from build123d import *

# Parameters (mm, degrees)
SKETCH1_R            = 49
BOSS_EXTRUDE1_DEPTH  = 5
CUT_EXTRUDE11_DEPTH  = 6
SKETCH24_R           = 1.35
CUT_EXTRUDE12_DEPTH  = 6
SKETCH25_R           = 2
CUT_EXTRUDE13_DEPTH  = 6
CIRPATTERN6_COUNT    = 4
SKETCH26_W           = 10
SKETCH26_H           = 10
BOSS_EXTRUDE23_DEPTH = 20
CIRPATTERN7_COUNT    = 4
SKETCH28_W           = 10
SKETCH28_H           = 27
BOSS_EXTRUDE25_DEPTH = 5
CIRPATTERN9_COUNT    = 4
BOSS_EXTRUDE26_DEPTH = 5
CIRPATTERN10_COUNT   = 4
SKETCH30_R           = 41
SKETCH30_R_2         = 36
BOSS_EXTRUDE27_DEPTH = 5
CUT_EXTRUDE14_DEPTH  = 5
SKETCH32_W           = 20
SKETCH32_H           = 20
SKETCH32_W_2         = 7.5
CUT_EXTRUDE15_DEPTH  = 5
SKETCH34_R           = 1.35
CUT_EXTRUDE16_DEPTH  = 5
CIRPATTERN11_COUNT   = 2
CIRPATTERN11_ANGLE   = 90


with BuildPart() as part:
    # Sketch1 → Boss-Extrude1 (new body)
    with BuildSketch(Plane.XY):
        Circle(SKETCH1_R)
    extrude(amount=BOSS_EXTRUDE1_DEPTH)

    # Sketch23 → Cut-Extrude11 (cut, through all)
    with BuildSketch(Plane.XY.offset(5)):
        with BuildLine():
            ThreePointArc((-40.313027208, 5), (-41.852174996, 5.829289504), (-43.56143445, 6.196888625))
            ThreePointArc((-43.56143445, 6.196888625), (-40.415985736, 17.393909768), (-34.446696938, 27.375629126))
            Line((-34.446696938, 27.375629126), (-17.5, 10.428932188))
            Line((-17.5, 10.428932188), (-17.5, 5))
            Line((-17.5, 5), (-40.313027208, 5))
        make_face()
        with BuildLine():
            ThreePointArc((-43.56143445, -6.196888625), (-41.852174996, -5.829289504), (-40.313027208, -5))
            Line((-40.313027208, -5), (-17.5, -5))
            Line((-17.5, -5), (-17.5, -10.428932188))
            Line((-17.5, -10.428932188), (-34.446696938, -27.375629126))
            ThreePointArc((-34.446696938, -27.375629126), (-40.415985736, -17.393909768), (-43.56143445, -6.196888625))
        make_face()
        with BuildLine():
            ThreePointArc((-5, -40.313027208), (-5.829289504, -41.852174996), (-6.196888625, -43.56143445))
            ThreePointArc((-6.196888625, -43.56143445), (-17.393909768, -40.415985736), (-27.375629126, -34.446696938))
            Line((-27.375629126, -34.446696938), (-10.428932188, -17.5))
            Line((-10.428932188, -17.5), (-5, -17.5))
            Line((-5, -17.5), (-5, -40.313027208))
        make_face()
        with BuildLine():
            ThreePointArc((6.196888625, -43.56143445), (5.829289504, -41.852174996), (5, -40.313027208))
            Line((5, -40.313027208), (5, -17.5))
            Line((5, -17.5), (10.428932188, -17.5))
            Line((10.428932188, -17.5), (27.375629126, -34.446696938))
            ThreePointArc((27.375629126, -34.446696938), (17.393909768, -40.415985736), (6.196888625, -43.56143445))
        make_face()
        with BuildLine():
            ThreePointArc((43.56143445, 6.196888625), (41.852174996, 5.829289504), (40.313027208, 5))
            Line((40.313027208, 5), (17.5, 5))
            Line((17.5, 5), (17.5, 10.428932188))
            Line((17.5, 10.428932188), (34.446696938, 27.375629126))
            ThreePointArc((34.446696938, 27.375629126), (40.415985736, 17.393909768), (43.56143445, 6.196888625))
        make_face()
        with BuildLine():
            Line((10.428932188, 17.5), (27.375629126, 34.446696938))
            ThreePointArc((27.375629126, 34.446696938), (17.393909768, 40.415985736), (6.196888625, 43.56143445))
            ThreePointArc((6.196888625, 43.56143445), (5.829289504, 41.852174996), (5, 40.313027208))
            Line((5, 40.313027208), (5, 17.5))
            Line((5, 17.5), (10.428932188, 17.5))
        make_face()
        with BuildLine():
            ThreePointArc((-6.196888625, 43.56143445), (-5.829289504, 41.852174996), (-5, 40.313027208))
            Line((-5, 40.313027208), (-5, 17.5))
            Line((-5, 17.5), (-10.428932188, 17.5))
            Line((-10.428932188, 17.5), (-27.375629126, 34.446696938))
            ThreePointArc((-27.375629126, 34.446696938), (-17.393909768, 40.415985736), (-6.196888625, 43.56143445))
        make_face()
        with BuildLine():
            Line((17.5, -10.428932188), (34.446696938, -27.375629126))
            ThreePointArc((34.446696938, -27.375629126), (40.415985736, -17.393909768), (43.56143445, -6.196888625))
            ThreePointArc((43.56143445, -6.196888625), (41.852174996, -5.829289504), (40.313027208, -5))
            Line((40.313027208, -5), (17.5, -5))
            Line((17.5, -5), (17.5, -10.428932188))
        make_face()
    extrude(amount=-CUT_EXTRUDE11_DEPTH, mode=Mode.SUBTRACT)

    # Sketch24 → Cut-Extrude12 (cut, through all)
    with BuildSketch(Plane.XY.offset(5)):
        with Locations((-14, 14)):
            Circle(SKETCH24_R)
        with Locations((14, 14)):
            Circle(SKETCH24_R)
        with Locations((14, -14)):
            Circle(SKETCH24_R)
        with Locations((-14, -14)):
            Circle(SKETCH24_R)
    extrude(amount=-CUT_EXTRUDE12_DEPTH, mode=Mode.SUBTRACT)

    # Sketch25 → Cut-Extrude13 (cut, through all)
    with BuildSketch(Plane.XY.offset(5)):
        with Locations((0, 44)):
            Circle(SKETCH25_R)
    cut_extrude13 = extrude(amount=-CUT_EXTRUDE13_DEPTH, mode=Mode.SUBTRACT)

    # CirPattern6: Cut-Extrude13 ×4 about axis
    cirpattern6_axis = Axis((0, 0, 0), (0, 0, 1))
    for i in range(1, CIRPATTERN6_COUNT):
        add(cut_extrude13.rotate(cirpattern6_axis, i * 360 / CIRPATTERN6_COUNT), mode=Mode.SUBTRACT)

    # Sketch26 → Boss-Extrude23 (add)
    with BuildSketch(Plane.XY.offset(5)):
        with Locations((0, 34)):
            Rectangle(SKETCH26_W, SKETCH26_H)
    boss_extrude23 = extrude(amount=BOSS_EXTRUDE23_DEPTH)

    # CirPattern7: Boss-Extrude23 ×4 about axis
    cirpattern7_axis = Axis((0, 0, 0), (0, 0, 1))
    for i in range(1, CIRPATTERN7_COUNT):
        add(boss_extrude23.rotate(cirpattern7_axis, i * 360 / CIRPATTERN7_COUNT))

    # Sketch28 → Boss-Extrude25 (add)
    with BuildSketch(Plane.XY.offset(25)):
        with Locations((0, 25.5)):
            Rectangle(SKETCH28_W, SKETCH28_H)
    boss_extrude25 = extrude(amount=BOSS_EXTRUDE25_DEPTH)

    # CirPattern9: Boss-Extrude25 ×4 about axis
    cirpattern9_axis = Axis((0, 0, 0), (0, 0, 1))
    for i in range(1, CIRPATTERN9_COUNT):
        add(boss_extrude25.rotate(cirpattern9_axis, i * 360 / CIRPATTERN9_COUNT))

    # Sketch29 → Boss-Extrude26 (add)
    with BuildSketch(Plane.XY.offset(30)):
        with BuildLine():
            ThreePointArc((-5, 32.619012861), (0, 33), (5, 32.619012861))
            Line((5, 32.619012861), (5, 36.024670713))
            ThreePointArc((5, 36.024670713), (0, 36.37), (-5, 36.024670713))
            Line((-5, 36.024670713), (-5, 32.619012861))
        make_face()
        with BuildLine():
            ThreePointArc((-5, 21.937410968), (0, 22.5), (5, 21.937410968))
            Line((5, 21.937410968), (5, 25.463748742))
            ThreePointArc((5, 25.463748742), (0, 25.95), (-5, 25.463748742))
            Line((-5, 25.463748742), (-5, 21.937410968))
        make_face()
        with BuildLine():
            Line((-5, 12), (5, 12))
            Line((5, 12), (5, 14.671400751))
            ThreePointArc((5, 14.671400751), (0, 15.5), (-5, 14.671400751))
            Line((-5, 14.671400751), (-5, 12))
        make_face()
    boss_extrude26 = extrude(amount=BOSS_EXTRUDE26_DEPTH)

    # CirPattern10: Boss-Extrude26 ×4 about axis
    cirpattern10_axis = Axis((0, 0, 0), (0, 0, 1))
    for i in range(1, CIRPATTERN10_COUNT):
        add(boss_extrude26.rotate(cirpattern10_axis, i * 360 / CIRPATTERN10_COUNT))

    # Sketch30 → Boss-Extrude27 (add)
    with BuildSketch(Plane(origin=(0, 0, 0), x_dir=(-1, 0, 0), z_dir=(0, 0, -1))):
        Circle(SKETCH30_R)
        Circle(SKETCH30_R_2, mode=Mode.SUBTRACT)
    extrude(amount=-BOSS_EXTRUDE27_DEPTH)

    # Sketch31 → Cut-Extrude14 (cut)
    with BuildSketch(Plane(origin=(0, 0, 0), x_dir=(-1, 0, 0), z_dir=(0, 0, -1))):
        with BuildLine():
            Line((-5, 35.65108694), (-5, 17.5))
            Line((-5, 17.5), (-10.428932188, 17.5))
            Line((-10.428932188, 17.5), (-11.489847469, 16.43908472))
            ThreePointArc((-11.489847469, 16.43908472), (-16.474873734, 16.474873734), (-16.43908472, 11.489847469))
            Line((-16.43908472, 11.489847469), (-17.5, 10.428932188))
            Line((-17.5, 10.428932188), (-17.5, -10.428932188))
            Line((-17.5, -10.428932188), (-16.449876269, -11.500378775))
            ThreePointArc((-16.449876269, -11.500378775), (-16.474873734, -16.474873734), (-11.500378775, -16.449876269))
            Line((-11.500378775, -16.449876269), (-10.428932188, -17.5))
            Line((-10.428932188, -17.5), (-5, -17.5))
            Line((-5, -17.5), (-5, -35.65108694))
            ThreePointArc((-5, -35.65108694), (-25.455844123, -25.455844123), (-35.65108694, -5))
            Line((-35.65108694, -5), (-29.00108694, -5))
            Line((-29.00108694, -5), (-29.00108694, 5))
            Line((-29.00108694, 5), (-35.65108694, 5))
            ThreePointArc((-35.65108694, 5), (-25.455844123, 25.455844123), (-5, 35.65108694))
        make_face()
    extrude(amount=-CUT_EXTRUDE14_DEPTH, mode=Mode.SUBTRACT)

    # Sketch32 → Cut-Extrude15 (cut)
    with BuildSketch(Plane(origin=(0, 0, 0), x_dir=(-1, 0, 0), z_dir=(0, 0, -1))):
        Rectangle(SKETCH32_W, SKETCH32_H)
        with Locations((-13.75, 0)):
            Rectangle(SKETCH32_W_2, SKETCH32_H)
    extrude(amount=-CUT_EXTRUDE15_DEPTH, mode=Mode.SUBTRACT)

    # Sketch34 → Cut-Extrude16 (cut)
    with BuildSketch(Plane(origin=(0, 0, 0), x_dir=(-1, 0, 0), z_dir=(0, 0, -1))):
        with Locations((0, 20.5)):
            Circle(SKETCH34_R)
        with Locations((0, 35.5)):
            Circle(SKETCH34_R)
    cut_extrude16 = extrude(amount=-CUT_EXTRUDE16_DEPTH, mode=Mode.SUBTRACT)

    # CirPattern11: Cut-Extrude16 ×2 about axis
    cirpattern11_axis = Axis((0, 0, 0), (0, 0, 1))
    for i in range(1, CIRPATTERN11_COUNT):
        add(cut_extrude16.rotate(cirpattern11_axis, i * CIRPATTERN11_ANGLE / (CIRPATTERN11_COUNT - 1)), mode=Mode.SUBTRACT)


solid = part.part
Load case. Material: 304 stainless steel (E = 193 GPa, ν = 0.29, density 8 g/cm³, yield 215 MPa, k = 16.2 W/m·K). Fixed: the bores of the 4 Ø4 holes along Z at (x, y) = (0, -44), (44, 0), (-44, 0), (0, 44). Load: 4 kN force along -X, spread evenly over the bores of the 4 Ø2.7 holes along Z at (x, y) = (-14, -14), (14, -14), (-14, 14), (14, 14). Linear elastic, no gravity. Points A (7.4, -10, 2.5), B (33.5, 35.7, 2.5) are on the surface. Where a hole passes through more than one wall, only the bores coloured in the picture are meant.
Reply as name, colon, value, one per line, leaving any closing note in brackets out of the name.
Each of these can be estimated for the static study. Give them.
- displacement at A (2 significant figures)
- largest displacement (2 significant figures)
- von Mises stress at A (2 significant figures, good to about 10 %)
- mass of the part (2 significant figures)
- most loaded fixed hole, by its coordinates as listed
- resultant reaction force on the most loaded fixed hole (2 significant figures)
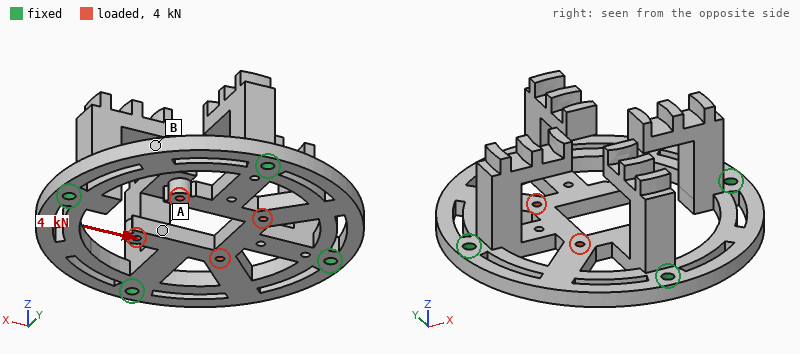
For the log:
displacement at A: 16 µm
largest displacement: 17 µm
von Mises stress at A: 21 MPa
mass of the part: 300 g
most loaded fixed hole, by its coordinates as listed: (-44, 0)
resultant reaction force on the most loaded fixed hole: 1.9 kN
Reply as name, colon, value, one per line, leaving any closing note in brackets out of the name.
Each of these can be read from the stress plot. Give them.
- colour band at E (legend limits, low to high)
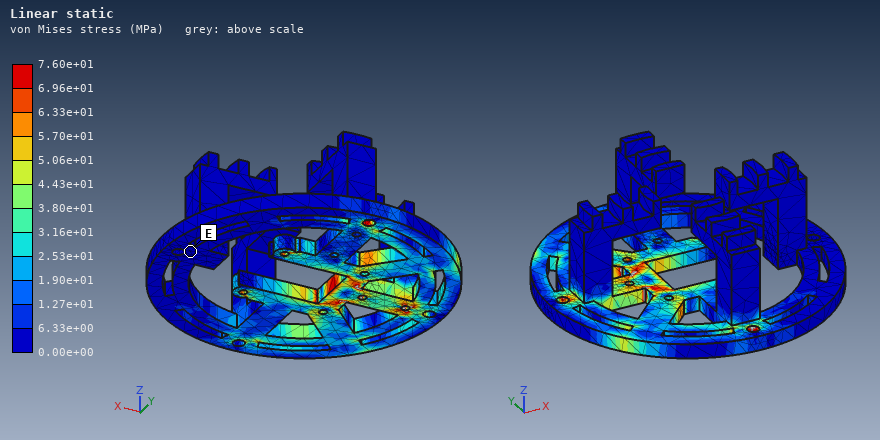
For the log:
colour band at E: 0.00e+00 to 6.33e+00 MPa
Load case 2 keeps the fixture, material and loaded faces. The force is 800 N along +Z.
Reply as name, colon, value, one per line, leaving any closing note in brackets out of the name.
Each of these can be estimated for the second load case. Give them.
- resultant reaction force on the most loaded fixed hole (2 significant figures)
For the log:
resultant reaction force on the most loaded fixed hole: 290 N
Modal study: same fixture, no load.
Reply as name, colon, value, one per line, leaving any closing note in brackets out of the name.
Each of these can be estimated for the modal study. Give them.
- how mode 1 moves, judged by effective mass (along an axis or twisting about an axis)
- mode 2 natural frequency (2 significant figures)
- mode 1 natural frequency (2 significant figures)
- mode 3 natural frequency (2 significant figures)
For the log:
how mode 1 moves, judged by effective mass: along Z
mode 2 natural frequency: 2100 Hz
mode 1 natural frequency: 1900 Hz
mode 3 natural frequency: 2400 Hz
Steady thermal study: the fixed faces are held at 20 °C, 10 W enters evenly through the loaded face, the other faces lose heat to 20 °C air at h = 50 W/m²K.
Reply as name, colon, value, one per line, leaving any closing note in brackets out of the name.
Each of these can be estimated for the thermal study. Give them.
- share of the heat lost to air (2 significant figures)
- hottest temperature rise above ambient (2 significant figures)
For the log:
share of the heat lost to air: 79 %
hottest temperature rise above ambient: 72 K
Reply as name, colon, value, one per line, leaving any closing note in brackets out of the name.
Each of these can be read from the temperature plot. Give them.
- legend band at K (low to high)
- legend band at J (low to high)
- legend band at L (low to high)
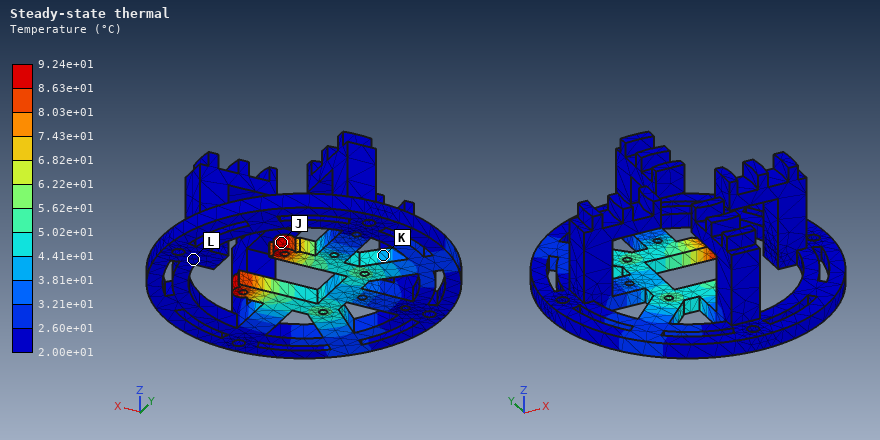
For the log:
legend band at K: 3.81e+01 to 4.41e+01 °C
legend band at J: 8.63e+01 to 9.24e+01 °C
legend band at L: 2.00e+01 to 2.60e+01 °C
